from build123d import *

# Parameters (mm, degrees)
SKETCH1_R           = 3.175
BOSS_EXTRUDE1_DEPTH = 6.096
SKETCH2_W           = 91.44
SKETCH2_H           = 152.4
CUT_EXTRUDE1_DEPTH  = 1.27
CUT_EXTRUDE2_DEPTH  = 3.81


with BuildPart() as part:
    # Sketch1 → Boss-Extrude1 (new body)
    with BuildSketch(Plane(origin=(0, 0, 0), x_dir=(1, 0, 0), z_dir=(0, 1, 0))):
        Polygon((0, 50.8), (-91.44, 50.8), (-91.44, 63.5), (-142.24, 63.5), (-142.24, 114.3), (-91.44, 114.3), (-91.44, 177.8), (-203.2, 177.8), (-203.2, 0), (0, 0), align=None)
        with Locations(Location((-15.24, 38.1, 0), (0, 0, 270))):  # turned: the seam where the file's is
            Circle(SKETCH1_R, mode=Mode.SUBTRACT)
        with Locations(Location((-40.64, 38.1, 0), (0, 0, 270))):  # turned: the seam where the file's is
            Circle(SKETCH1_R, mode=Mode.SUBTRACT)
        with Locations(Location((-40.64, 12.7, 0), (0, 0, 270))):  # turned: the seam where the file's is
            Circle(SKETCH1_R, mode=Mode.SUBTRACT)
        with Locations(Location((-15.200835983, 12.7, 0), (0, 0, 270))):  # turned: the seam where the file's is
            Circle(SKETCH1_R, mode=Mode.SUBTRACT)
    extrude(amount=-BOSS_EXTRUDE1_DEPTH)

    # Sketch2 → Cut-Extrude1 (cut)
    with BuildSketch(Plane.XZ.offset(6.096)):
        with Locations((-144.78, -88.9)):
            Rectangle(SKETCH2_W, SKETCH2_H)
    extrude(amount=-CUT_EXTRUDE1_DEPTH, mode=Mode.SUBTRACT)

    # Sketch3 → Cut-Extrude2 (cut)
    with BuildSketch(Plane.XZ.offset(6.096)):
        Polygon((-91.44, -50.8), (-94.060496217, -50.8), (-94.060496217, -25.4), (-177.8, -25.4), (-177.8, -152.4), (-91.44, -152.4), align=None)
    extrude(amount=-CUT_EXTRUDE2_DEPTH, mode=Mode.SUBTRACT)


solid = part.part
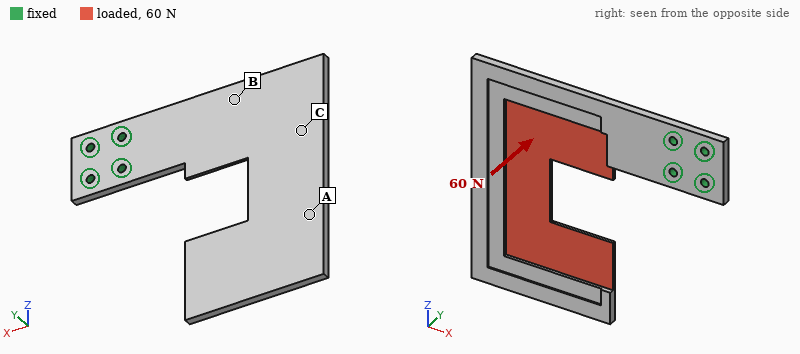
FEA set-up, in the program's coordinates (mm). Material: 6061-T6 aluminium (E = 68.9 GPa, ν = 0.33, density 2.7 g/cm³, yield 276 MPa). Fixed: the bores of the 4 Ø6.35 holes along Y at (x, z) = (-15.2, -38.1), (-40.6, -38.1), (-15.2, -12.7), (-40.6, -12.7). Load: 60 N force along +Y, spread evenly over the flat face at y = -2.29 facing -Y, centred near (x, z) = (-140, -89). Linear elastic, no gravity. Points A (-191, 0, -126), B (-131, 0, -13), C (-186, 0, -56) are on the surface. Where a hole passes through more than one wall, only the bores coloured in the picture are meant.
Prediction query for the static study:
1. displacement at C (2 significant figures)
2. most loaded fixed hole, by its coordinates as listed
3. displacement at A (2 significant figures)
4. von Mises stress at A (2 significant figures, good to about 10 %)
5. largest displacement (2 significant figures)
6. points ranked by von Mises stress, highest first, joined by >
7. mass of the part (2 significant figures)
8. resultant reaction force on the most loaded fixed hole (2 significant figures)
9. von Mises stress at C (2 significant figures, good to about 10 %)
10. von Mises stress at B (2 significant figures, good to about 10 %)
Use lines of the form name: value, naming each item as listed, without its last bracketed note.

displacement at C: 0.98 mm
most loaded fixed hole, by its coordinates as listed: (-40.6, -38.1)
displacement at A: 2.0 mm
von Mises stress at A: 5.8 MPa
largest displacement: 2.8 mm
points ranked by von Mises stress, highest first, joined by >: B > C > A
mass of the part: 260 g
resultant reaction force on the most loaded fixed hole: 180 N
von Mises stress at C: 13 MPa
von Mises stress at B: 22 MPa
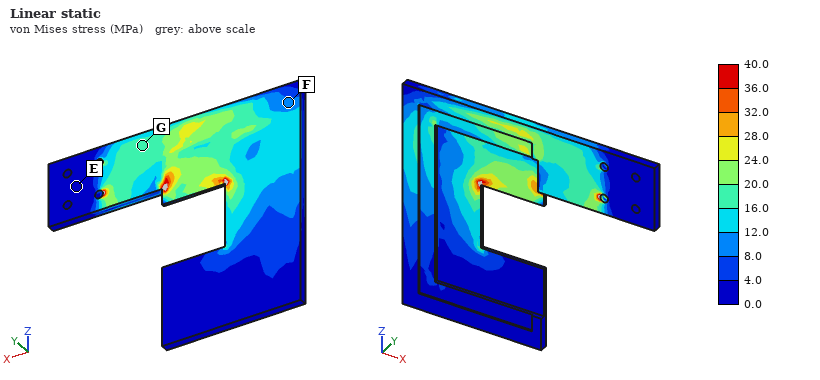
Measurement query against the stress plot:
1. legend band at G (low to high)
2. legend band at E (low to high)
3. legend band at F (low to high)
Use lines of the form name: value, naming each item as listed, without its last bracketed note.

legend band at G: 16.0 to 20.0 MPa
legend band at E: 0.0 to 4.0 MPa
legend band at F: 8.0 to 12.0 MPa
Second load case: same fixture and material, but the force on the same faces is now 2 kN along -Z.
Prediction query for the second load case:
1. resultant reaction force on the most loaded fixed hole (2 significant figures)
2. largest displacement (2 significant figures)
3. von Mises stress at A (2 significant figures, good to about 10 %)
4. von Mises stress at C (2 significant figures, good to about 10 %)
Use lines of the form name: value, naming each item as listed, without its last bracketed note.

resultant reaction force on the most loaded fixed hole: 5.4 kN
largest displacement: 1.4 mm
von Mises stress at A: 11 MPa
von Mises stress at C: 10 MPa
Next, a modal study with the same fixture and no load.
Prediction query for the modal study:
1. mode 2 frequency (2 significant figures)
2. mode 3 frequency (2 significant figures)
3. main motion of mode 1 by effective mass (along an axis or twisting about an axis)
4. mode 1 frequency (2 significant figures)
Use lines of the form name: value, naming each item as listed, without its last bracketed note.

mode 2 frequency: 130 Hz
mode 3 frequency: 310 Hz
main motion of mode 1 by effective mass: along Y
mode 1 frequency: 60 Hz
